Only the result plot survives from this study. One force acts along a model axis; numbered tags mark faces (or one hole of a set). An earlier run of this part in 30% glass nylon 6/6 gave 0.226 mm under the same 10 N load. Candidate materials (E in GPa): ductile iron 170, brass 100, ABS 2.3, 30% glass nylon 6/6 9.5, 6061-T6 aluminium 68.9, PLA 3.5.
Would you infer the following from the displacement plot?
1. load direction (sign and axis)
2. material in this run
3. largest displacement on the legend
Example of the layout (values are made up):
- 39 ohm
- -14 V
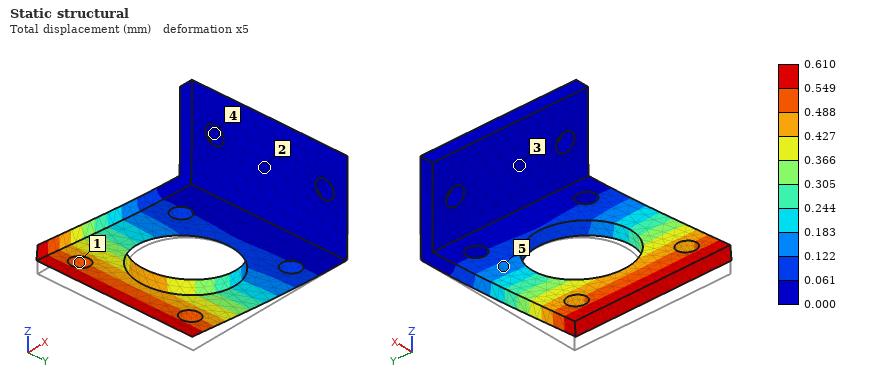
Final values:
- +Z
- PLA
- 0.610 mm
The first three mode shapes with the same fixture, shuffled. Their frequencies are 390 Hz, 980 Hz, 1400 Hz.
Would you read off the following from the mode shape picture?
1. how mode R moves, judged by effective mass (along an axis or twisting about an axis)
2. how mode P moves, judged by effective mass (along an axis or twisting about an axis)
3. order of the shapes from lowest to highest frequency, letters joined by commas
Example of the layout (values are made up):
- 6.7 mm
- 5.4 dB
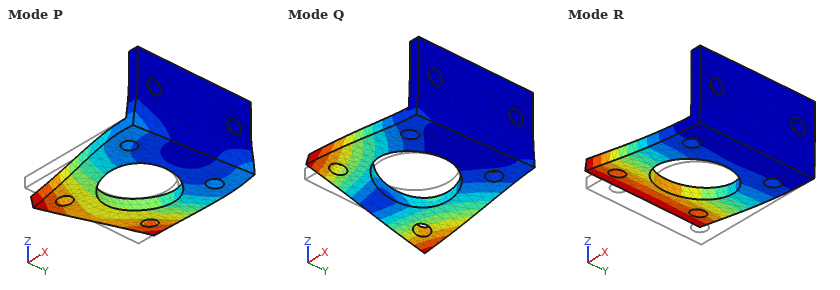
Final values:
- along Z
- along Y
- R, Q, P
